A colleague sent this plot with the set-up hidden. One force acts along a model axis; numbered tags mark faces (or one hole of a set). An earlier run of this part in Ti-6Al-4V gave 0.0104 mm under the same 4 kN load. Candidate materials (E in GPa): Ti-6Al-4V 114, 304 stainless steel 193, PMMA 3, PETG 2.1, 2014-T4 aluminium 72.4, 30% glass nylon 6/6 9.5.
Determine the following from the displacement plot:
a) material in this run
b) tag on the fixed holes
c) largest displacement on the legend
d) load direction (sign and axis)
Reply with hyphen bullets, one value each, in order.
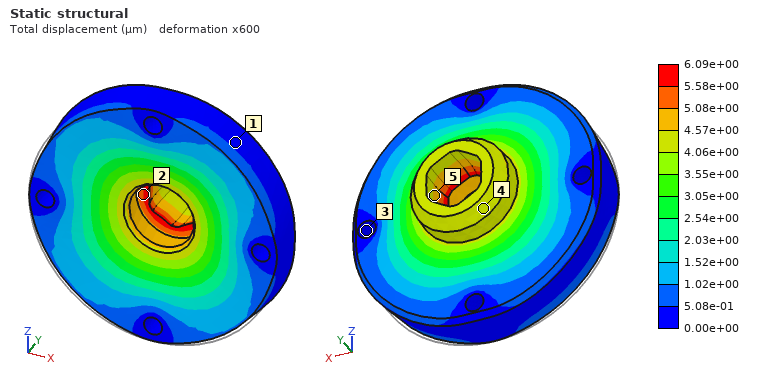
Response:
- 304 stainless steel
- 3
- 6.09e+00 µm
- +Y
